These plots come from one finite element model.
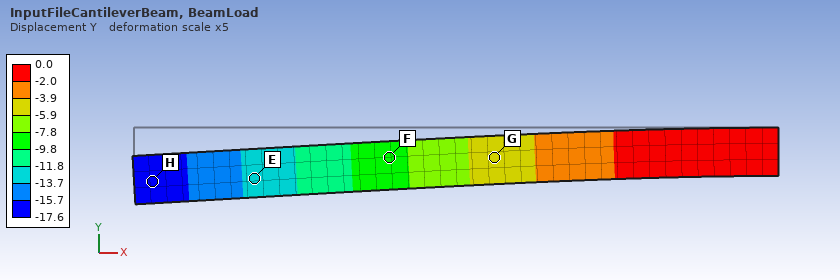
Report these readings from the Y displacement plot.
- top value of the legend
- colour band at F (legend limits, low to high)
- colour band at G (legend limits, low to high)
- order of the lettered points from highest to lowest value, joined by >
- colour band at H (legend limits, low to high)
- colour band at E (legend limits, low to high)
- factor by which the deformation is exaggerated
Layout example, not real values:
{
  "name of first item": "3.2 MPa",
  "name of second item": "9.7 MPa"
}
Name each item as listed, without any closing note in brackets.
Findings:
{
  "top value of the legend": "0.0",
  "colour band at F": "-9.8 to -7.8",
  "colour band at G": "-5.9 to -3.9",
  "order of the lettered points from highest to lowest value, joined by >": "G > F > E > H",
  "colour band at H": "-17.6 to -15.7",
  "colour band at E": "-13.7 to -11.8",
  "factor by which the deformation is exaggerated": "5"
}
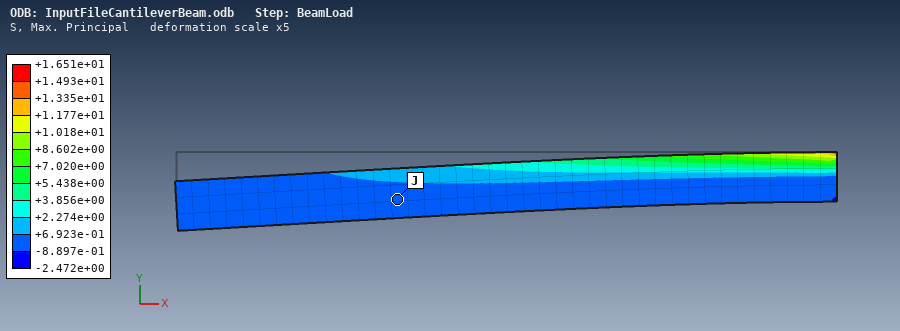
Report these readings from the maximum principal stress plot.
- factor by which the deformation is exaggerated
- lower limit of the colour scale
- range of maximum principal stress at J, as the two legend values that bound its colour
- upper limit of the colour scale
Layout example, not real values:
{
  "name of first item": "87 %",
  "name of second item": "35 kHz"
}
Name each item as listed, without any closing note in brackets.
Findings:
{
  "factor by which the deformation is exaggerated": "5",
  "lower limit of the colour scale": "-2.472e+00",
  "range of maximum principal stress at J, as the two legend values that bound its colour": "-8.897e-01 to +6.923e-01",
  "upper limit of the colour scale": "+1.651e+01"
}
